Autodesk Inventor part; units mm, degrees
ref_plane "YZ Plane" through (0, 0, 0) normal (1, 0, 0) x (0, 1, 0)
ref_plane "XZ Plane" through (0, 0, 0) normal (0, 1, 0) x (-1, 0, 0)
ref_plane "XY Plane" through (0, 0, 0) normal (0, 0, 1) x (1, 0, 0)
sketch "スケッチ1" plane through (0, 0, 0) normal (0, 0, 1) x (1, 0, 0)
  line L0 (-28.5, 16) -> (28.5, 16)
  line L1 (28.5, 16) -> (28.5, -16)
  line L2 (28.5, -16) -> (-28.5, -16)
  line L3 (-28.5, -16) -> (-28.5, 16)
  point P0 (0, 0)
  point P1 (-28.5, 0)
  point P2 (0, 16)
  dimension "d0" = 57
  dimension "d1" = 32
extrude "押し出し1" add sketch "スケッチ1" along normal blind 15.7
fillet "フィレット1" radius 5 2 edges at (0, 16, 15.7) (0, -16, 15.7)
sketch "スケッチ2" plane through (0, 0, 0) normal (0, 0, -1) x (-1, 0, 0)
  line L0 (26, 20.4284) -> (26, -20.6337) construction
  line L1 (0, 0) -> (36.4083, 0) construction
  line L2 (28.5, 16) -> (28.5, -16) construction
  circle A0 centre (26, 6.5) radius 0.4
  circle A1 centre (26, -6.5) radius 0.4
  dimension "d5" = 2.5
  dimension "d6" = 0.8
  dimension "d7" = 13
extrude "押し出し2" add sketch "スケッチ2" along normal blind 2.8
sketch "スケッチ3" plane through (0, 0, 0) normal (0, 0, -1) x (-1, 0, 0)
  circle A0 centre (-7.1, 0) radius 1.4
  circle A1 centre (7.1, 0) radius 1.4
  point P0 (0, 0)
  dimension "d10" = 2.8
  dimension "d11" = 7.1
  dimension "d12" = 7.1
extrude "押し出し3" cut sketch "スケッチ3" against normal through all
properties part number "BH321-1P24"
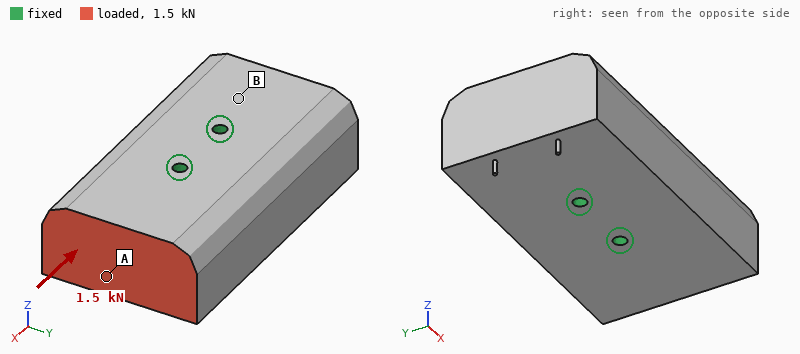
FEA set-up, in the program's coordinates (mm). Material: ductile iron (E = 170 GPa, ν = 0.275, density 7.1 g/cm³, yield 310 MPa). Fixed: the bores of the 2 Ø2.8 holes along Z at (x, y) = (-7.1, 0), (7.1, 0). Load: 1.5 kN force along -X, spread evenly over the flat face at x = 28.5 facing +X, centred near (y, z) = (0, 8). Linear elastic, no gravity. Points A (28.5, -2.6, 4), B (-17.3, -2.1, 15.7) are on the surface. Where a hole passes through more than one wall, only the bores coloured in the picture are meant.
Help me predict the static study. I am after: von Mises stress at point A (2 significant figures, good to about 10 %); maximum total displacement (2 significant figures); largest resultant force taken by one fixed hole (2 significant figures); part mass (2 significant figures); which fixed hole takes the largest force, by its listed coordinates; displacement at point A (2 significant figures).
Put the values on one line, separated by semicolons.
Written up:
3.5 MPa; 0.60 µm; 1.0 kN; 200 g; (7.1, 0); 0.55 µm
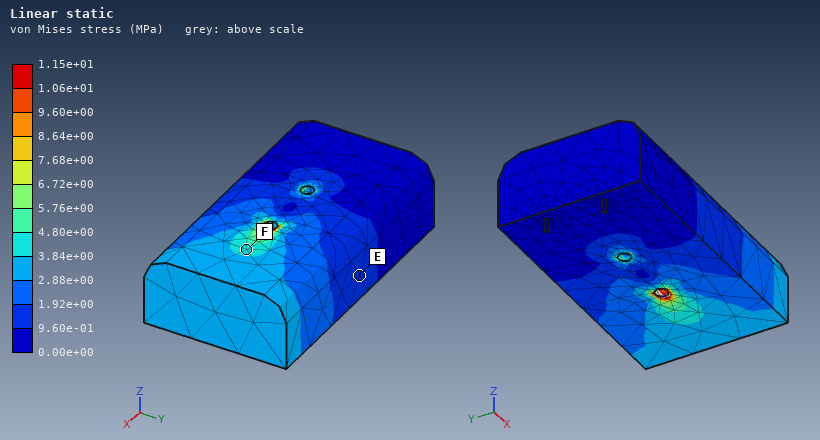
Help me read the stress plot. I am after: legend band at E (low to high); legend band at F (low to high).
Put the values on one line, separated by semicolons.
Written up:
9.60e-01 to 1.92e+00 MPa; 3.84e+00 to 4.80e+00 MPa
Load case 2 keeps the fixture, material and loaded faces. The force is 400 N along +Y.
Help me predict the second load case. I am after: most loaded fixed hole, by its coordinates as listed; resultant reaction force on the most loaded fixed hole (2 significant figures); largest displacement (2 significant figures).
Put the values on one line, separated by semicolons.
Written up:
(7.1, 0); 910 N; 1.6 µm
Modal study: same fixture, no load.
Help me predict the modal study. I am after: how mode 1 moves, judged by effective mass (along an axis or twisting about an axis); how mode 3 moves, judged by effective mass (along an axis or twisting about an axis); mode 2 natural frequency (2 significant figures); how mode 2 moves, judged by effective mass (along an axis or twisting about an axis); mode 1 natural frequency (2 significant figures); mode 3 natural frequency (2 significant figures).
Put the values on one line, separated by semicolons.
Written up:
twisting about Z; along Z; 14 kHz; twisting about Y; 12 kHz; 16 kHz
